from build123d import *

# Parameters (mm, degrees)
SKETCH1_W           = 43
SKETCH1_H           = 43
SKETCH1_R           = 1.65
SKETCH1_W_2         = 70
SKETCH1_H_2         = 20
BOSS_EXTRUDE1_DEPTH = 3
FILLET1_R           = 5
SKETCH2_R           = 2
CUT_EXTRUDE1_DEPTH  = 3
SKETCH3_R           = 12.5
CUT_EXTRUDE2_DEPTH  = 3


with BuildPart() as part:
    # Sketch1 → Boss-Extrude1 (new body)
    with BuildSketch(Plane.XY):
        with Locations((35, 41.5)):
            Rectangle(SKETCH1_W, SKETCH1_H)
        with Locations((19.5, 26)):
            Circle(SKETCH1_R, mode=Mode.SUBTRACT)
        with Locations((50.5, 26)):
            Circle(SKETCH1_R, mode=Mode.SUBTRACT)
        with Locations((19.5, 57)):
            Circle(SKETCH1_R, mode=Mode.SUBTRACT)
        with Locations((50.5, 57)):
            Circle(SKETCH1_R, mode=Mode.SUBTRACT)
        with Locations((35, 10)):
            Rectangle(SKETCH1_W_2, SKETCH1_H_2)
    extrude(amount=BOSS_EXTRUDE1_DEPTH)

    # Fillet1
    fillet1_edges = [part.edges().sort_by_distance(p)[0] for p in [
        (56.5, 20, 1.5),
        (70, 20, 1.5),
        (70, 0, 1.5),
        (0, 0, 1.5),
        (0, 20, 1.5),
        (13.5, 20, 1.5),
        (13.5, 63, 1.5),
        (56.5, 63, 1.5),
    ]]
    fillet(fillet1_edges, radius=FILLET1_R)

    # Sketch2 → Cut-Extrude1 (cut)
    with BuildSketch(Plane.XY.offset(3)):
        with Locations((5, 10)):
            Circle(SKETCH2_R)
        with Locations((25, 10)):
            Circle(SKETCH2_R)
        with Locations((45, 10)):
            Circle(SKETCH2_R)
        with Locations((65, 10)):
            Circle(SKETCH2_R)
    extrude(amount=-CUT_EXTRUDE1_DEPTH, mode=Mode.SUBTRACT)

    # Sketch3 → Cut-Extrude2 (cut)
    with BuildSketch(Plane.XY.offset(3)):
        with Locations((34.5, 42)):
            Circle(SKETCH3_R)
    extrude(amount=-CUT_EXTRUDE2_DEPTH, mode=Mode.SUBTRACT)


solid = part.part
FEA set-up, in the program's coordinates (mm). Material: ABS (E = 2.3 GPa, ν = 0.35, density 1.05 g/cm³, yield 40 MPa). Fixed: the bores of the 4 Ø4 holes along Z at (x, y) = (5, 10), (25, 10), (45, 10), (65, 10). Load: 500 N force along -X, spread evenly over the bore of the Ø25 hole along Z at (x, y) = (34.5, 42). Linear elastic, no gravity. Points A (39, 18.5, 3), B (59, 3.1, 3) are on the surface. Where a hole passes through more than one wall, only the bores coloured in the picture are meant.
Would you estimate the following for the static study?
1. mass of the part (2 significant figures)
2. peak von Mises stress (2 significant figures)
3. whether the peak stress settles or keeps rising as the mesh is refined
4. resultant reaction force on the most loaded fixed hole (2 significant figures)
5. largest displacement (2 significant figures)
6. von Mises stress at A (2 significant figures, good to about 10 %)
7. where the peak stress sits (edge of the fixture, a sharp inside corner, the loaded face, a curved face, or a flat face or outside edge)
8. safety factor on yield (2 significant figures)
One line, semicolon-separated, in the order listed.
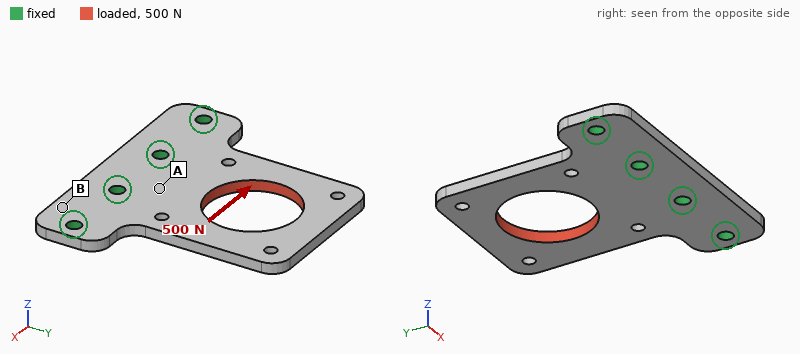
8.4 g; 33 MPa; settles; 240 N; 0.80 mm; 8.6 MPa; a curved face; 1.2
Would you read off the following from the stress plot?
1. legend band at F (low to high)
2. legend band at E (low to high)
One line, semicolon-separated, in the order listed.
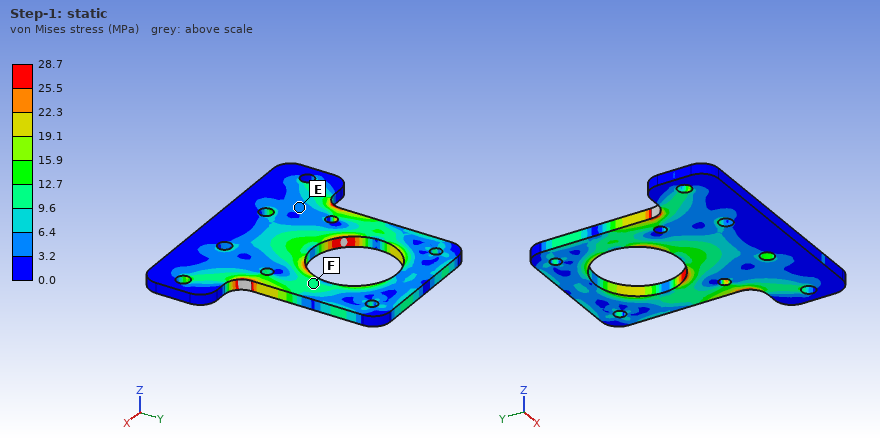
9.6 to 12.7 MPa; 3.2 to 6.4 MPa
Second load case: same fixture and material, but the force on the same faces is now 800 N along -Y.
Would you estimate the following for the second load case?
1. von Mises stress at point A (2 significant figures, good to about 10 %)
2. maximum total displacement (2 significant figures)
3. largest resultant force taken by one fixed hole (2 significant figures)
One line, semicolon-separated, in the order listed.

3.0 MPa; 0.29 mm; 290 N
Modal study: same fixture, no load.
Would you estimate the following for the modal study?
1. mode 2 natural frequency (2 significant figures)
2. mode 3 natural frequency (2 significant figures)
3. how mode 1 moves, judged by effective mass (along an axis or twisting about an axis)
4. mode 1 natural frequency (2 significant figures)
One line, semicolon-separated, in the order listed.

690 Hz; 1600 Hz; along Z; 280 Hz
